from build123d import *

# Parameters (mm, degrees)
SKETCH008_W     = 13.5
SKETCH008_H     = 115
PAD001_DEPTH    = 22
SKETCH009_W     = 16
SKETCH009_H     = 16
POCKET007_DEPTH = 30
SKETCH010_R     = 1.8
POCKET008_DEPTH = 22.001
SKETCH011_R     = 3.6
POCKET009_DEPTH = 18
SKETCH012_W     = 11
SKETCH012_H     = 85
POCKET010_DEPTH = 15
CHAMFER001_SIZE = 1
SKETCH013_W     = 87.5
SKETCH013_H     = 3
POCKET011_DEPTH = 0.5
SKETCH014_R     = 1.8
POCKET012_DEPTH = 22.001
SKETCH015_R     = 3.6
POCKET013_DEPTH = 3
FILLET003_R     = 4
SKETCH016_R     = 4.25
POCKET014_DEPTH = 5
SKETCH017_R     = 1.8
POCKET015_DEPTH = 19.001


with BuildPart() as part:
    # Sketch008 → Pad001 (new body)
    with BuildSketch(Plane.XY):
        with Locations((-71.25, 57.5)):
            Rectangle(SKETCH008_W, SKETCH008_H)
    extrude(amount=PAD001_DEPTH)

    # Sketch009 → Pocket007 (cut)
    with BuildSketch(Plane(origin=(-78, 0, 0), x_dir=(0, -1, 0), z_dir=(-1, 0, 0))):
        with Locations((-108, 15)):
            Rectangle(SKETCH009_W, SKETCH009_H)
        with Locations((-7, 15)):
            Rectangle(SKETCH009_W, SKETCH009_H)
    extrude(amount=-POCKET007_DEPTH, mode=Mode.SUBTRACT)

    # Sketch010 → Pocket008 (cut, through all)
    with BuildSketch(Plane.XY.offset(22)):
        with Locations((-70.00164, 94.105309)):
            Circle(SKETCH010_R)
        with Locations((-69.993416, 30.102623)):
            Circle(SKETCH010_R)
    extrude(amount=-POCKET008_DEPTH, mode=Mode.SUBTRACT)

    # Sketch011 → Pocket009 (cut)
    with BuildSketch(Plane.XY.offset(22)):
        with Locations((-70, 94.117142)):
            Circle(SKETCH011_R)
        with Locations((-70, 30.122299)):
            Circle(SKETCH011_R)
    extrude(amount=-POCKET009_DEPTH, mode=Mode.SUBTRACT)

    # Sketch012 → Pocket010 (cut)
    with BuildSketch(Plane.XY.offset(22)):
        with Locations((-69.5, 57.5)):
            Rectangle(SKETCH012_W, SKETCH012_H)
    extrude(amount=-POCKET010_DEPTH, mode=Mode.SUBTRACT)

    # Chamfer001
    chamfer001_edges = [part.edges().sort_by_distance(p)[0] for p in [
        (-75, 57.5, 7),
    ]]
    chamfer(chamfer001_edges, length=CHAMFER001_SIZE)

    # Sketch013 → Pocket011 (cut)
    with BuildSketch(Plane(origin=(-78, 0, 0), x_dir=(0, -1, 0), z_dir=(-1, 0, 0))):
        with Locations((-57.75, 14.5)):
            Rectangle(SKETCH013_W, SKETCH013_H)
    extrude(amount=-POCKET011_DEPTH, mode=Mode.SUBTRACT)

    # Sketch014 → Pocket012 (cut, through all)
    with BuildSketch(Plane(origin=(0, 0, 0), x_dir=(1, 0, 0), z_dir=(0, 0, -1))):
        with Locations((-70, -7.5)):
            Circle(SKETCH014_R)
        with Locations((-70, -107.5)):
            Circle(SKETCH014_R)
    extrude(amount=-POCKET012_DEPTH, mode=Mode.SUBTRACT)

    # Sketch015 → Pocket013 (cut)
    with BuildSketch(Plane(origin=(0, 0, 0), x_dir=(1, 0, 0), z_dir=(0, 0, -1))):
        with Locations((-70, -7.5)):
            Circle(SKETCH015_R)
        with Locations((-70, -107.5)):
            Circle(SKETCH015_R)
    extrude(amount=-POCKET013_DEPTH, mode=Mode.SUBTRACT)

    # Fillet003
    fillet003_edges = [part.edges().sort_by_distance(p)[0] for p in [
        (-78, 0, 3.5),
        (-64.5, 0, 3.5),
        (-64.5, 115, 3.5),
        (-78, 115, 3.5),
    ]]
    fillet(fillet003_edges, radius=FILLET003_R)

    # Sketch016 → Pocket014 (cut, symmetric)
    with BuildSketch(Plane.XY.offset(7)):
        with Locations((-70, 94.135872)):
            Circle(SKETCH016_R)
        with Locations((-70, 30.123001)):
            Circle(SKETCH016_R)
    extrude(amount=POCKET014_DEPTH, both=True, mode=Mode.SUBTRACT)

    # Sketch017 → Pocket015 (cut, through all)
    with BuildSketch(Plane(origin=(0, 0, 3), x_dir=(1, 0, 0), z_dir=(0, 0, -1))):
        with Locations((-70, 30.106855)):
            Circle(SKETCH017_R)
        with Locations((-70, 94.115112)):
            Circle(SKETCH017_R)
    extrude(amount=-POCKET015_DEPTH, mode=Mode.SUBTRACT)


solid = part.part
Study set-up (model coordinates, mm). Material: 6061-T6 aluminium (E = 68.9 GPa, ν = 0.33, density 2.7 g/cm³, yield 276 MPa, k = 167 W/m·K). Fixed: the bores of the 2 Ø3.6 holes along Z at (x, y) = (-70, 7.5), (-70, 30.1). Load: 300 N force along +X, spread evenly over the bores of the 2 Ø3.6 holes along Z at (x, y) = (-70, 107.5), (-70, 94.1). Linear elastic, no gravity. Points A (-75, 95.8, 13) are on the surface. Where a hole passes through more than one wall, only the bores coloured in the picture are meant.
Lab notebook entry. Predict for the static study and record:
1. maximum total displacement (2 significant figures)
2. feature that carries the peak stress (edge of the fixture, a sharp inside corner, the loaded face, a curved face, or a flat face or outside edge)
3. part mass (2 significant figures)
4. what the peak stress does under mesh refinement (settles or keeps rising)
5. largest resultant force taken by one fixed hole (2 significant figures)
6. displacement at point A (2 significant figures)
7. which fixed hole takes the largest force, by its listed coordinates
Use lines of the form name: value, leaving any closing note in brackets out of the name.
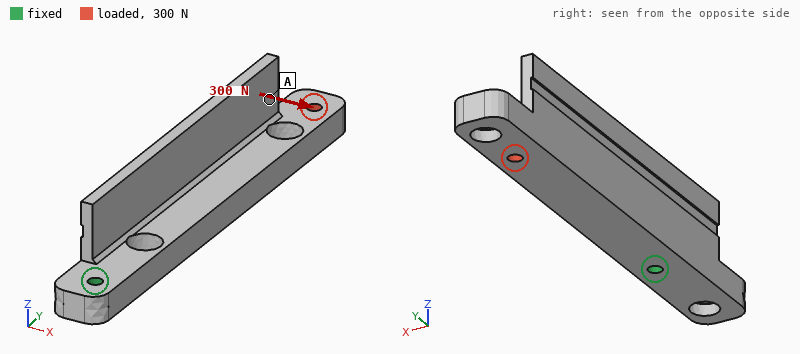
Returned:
maximum total displacement: 0.69 mm
feature that carries the peak stress: edge of the fixture
part mass: 37 g
what the peak stress does under mesh refinement: keeps rising
largest resultant force taken by one fixed hole: 1.1 kN
displacement at point A: 0.50 mm
which fixed hole takes the largest force, by its listed coordinates: (-70, 30.1)
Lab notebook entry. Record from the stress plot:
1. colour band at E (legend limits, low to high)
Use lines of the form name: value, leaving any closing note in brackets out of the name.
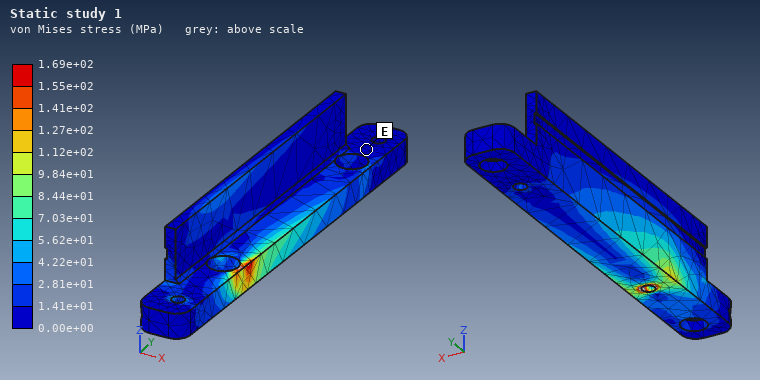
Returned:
colour band at E: 0.00e+00 to 1.41e+01 MPa
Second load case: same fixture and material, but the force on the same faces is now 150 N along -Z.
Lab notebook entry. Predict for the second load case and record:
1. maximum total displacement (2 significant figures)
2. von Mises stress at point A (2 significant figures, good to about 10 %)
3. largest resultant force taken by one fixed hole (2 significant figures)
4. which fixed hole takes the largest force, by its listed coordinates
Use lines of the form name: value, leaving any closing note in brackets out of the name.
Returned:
maximum total displacement: 0.28 mm
von Mises stress at point A: 10 MPa
largest resultant force taken by one fixed hole: 700 N
which fixed hole takes the largest force, by its listed coordinates: (-70, 30.1)
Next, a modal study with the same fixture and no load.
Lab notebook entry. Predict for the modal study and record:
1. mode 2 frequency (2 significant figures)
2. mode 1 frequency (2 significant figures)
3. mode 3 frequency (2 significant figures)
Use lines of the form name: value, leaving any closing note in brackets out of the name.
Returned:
mode 2 frequency: 1600 Hz
mode 1 frequency: 1100 Hz
mode 3 frequency: 3200 Hz
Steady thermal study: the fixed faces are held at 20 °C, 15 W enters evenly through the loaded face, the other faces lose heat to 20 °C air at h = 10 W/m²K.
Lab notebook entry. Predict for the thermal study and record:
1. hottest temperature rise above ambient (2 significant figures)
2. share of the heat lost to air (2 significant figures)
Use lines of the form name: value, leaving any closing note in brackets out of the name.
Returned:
hottest temperature rise above ambient: 60 K
share of the heat lost to air: 13 %
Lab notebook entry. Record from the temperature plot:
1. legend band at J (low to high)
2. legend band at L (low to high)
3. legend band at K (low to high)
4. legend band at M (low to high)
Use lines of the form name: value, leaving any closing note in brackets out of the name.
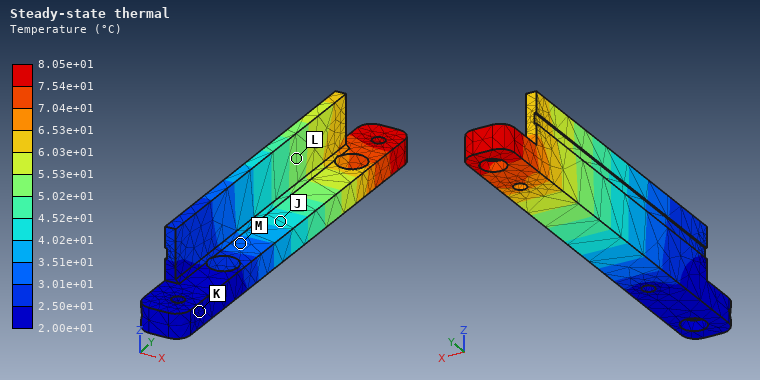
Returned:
legend band at J: 4.02e+01 to 4.52e+01 °C
legend band at L: 5.02e+01 to 5.53e+01 °C
legend band at K: 2.00e+01 to 2.50e+01 °C
legend band at M: 3.01e+01 to 3.51e+01 °C
